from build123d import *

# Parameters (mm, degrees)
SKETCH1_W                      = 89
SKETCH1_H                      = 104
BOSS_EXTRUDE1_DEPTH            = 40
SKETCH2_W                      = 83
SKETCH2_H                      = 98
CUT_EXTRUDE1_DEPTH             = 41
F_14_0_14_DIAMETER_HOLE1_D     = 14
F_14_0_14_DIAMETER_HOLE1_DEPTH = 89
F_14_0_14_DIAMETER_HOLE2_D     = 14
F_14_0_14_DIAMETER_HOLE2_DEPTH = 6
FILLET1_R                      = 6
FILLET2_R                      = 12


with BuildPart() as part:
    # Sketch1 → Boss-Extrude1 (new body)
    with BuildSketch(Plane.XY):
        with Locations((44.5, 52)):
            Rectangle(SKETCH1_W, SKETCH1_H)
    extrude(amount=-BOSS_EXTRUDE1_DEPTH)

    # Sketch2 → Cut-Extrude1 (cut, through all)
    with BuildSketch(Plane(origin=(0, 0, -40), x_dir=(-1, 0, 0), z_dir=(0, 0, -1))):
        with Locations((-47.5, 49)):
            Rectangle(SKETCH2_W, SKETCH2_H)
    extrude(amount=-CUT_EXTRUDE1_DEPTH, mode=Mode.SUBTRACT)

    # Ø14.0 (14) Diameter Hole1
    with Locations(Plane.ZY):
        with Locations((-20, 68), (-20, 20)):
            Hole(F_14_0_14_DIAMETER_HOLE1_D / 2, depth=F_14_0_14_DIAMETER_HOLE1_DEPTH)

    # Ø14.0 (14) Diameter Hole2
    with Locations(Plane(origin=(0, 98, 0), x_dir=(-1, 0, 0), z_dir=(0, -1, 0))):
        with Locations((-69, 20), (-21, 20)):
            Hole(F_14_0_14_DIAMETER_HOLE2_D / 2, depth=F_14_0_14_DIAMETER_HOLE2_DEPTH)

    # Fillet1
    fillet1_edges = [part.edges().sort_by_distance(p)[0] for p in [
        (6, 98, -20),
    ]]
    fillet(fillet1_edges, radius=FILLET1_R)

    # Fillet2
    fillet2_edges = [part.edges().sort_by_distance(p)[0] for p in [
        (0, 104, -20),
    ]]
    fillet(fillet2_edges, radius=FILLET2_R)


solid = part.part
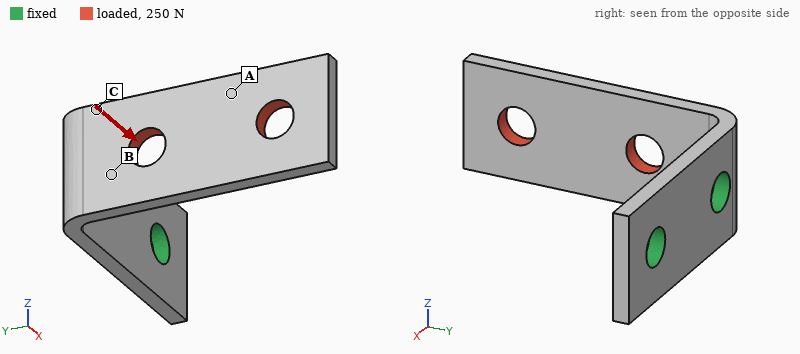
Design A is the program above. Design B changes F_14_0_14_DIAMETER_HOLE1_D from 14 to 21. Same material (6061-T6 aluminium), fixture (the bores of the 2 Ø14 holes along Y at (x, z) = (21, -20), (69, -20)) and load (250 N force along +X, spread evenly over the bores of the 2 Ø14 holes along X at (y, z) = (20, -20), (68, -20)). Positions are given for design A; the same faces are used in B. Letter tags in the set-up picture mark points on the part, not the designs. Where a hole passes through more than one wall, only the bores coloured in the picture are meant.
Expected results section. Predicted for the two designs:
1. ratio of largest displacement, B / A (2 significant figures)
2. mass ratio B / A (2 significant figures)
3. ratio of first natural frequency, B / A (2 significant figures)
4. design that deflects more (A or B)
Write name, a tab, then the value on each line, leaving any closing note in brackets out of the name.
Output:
ratio of largest displacement, B / A	1.1
mass ratio B / A	0.94
ratio of first natural frequency, B / A	1.0
design that deflects more	B
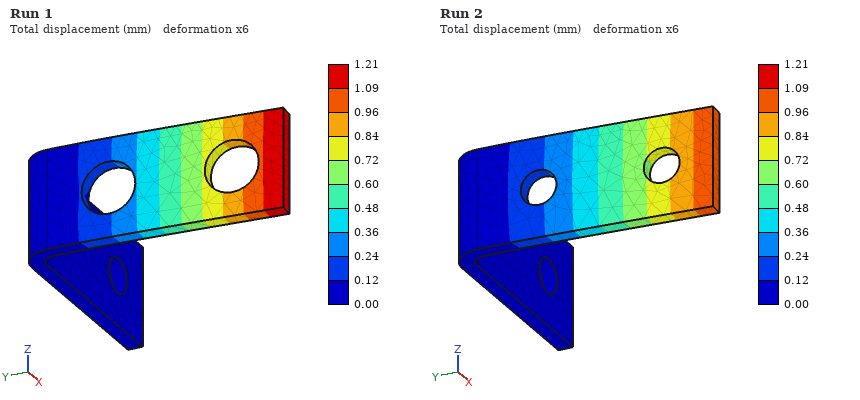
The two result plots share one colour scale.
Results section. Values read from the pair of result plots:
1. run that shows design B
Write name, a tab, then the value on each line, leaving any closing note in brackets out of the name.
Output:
run that shows design B	Run 1
